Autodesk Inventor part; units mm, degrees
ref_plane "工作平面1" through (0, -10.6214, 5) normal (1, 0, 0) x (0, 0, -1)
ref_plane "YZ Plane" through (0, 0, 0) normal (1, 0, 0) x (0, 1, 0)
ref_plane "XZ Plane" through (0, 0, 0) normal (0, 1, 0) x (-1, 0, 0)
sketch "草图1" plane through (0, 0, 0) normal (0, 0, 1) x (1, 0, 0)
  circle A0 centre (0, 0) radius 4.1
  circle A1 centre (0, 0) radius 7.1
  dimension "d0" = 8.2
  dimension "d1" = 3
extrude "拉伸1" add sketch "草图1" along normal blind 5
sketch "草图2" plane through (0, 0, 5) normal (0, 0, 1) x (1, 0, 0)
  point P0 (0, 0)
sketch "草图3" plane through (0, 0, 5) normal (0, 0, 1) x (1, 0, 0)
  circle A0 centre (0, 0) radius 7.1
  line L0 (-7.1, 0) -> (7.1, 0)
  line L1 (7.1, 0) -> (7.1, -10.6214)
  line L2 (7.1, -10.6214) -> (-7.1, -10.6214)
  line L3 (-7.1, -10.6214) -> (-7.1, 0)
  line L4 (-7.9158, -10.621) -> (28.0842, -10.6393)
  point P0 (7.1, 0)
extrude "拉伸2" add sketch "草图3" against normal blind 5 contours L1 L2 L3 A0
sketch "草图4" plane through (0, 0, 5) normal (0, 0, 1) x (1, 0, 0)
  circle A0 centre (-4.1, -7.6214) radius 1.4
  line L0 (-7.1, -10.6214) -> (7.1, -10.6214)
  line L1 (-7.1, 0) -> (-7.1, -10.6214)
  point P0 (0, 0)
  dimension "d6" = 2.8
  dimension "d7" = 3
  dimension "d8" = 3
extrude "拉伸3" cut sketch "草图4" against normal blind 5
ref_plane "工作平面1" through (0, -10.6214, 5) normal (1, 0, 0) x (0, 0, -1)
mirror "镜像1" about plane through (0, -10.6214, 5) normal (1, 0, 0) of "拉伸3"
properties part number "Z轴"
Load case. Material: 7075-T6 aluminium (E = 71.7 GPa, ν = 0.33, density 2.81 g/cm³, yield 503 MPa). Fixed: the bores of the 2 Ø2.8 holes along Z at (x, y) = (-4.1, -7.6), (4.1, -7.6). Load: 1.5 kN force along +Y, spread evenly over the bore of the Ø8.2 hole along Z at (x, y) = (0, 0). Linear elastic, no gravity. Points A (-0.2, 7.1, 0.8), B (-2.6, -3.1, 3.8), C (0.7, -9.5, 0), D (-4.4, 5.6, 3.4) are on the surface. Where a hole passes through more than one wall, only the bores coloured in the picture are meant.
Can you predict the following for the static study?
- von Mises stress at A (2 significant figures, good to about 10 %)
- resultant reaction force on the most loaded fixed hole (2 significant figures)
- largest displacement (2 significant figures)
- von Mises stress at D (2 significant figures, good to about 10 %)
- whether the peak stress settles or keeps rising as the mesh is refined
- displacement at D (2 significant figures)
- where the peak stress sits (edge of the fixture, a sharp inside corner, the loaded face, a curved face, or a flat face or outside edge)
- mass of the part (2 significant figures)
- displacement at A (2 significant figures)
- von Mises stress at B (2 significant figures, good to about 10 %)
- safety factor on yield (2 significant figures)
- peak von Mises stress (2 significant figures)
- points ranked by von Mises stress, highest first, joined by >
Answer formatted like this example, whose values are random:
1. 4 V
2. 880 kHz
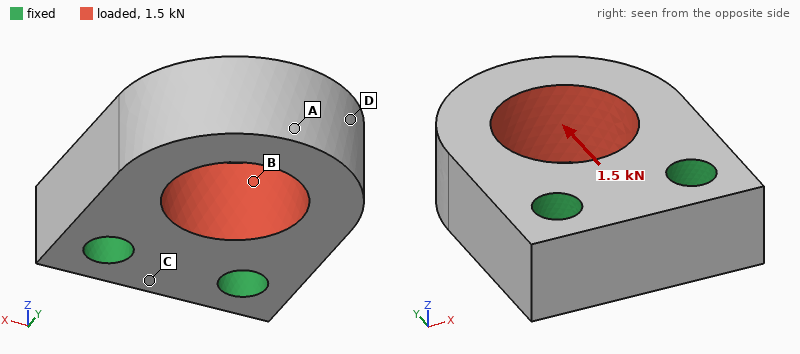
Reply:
1. 36 MPa
2. 750 N
3. 9.0 µm
4. 17 MPa
5. settles
6. 5.3 µm
7. the loaded face
8. 2.3 g
9. 8.4 µm
10. 24 MPa
11. 6.8
12. 74 MPa
13. A > B > D > C
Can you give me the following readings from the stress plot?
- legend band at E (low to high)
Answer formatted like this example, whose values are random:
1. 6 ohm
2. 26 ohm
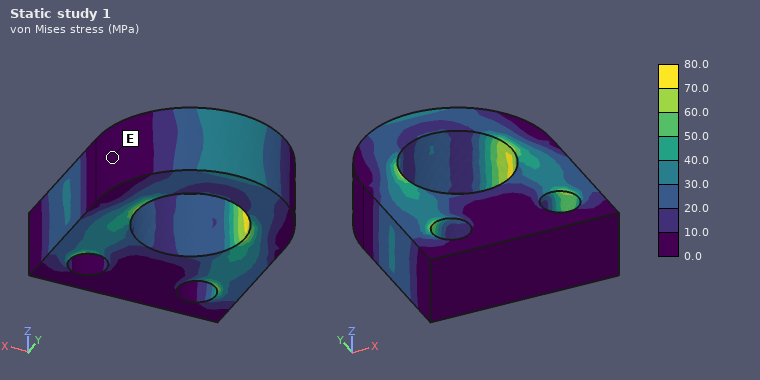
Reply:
1. 0.0 to 10.0 MPa
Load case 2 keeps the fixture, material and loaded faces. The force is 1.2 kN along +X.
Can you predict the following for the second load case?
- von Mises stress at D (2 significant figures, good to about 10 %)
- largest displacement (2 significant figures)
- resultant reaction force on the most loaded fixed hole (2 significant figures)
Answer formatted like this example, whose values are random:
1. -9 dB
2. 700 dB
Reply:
1. 49 MPa
2. 32 µm
3. 910 N
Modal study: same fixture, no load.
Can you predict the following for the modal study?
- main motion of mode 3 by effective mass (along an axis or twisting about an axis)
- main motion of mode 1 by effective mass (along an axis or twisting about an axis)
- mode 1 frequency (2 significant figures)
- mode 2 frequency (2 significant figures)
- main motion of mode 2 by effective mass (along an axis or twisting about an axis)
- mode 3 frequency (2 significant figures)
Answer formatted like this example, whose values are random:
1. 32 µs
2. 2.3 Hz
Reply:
1. twisting about Y
2. along Z
3. 20 kHz
4. 28 kHz
5. along X
6. 41 kHz
